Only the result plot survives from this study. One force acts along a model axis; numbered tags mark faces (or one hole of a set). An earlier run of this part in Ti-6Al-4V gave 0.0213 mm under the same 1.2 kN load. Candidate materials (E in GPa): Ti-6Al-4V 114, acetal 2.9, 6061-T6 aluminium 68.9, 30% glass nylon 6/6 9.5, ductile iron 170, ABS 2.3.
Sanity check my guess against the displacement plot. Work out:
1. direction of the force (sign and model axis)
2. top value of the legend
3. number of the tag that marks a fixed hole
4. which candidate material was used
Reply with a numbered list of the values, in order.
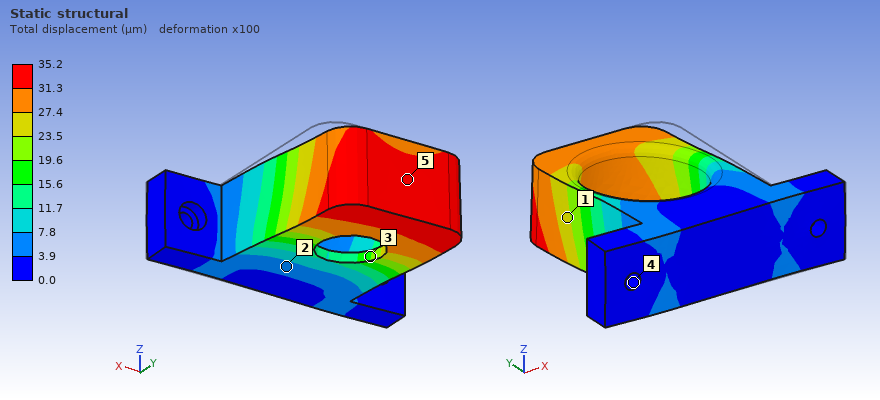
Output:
1. -X
2. 35.2 µm
3. 4
4. 6061-T6 aluminium
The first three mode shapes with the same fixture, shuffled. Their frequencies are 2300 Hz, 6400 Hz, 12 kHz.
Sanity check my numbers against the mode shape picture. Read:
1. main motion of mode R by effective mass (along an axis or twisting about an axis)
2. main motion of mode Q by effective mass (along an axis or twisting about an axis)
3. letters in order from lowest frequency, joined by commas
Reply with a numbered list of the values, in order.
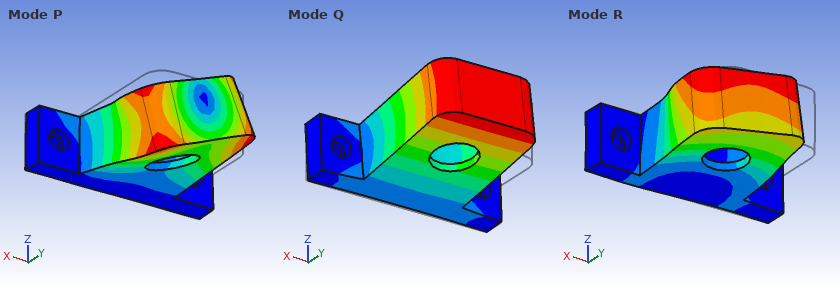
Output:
1. along X
2. along Z
3. Q, R, P
